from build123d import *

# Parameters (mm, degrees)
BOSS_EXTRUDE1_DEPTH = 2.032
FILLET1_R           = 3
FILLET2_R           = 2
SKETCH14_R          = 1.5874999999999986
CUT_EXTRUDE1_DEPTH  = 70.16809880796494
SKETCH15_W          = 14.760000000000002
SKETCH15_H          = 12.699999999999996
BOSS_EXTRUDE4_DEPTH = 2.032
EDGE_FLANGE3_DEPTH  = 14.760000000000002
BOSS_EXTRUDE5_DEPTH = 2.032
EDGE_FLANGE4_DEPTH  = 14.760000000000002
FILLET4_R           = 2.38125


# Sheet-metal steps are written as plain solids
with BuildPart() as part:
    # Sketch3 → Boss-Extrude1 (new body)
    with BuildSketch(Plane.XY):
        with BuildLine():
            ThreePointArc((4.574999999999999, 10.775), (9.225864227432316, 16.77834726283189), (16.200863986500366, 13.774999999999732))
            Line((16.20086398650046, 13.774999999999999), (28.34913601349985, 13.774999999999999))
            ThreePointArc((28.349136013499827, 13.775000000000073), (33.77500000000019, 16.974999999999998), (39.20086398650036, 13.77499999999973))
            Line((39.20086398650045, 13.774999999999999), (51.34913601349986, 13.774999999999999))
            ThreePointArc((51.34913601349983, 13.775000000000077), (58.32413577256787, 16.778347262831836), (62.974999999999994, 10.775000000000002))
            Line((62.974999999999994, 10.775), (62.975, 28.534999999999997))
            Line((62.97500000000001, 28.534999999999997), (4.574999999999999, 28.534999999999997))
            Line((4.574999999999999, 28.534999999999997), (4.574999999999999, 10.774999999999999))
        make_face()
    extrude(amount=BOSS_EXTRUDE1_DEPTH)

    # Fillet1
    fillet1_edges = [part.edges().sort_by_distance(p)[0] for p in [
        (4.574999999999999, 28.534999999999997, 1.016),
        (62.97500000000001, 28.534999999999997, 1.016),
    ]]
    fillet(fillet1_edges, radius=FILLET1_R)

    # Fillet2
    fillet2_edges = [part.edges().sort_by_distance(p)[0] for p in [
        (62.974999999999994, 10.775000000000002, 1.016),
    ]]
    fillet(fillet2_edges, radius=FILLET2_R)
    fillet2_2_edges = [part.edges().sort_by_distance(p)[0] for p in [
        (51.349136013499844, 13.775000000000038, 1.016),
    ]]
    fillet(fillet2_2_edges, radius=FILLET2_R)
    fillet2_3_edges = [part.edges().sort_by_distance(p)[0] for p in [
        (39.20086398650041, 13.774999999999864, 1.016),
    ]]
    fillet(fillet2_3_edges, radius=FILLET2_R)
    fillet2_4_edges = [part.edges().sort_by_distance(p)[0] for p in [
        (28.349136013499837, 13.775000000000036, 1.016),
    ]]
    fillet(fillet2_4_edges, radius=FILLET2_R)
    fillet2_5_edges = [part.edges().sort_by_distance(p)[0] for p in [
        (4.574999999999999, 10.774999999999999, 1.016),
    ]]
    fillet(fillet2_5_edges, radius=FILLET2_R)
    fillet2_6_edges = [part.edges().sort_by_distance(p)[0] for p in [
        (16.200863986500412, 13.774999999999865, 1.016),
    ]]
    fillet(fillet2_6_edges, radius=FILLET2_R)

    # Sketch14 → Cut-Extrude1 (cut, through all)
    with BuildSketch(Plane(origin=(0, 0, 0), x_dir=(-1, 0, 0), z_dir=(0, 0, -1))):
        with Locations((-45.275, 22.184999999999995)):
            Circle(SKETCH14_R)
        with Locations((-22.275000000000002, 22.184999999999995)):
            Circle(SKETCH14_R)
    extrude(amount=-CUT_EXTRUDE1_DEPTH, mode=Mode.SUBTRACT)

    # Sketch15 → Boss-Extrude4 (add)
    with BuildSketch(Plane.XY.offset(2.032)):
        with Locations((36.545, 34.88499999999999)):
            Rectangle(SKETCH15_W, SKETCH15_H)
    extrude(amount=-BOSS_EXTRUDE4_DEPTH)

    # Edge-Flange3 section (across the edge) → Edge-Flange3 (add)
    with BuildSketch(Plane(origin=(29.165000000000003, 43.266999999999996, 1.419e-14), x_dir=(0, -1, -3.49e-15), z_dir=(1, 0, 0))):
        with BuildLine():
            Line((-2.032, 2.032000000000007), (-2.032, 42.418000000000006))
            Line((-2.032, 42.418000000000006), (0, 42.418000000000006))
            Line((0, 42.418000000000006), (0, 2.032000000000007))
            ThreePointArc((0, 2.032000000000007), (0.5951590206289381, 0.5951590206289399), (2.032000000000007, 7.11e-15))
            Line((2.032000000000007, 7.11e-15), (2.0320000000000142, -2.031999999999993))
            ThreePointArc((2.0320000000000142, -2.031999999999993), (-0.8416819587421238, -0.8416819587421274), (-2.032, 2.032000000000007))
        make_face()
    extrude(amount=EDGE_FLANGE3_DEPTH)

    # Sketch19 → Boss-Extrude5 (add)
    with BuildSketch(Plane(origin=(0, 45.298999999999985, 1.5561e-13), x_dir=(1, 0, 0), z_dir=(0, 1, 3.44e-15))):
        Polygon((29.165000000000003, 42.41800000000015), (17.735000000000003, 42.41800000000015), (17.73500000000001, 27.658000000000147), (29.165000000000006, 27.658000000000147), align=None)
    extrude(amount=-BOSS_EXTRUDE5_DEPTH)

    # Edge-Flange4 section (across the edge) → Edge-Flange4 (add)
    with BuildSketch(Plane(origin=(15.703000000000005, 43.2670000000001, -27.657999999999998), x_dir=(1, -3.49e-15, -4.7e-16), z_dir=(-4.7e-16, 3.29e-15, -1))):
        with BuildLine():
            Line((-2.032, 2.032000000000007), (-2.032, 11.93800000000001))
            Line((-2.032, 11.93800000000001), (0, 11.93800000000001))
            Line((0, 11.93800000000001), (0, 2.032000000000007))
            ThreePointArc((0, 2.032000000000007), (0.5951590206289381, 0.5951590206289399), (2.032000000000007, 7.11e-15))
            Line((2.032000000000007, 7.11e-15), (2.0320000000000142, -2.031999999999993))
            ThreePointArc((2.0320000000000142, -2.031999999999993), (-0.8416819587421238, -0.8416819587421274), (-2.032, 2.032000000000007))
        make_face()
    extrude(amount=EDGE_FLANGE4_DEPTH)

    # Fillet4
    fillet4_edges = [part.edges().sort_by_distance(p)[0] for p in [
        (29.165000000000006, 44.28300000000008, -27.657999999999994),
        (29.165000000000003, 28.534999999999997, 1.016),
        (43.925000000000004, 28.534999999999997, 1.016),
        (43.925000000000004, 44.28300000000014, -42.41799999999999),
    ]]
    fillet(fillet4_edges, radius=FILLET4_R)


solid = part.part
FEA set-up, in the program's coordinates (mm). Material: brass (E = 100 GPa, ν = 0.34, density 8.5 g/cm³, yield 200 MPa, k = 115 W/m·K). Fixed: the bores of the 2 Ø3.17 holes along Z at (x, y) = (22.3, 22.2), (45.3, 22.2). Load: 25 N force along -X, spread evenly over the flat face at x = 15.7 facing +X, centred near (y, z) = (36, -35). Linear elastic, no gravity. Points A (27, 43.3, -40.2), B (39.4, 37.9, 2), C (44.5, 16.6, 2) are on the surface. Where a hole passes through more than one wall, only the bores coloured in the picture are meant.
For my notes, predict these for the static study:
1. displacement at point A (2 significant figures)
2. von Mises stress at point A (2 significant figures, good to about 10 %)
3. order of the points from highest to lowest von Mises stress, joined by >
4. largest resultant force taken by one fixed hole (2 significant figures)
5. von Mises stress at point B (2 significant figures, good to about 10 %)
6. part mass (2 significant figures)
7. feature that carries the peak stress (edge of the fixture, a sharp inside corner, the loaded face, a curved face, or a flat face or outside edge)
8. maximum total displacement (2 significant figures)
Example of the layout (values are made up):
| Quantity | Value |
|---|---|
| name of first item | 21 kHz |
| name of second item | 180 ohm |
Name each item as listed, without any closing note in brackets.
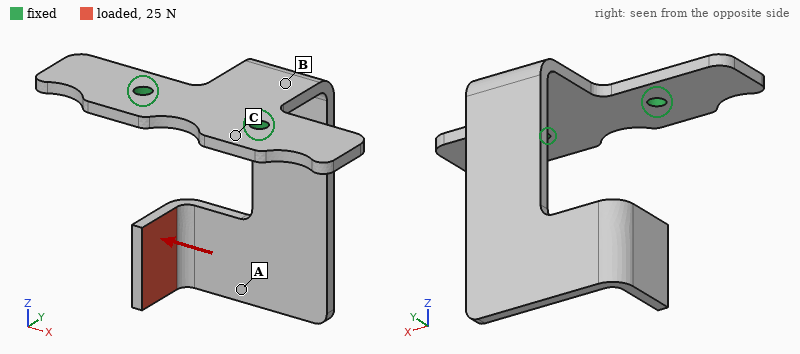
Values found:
| Quantity | Value |
|---|---|
| displacement at point A | 0.43 mm |
| von Mises stress at point A | 18 MPa |
| order of the points from highest to lowest von Mises stress, joined by > | B > A > C |
| largest resultant force taken by one fixed hole | 52 N |
| von Mises stress at point B | 73 MPa |
| part mass | 35 g |
| feature that carries the peak stress | a curved face |
| maximum total displacement | 0.62 mm |
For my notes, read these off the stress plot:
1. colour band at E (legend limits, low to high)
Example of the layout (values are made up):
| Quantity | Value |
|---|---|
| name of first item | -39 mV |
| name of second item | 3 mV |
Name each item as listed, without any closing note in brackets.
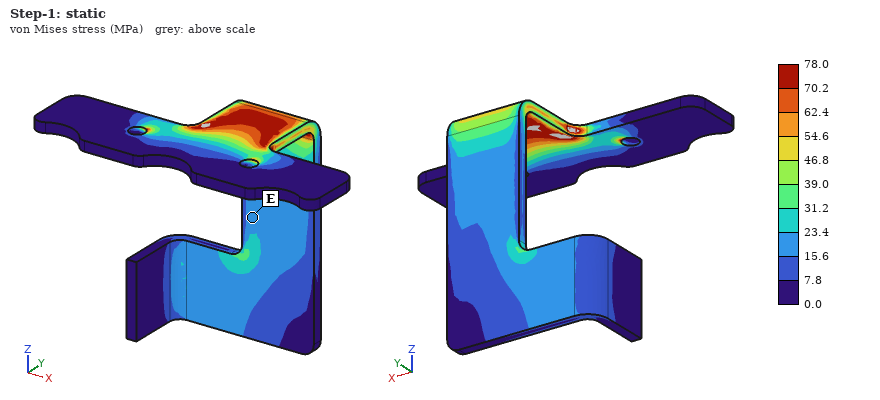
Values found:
| Quantity | Value |
|---|---|
| colour band at E | 15.6 to 23.4 MPa |
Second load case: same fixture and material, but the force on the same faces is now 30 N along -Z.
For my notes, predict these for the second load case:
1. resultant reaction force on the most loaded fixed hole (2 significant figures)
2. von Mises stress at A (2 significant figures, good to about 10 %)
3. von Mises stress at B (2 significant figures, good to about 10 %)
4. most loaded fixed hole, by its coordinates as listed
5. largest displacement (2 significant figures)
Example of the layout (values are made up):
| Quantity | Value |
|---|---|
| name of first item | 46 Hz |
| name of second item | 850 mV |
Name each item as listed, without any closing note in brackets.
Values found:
| Quantity | Value |
|---|---|
| resultant reaction force on the most loaded fixed hole | 44 N |
| von Mises stress at A | 16 MPa |
| von Mises stress at B | 49 MPa |
| most loaded fixed hole, by its coordinates as listed | (22.3, 22.2) |
| largest displacement | 0.45 mm |
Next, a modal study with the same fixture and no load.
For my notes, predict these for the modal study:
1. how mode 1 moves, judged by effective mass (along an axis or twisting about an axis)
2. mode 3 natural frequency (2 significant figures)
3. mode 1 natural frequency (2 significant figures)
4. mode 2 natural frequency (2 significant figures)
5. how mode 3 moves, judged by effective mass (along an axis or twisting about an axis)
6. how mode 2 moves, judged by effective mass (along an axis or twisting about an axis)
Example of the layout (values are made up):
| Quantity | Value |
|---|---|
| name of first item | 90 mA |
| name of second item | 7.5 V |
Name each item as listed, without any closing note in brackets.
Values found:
| Quantity | Value |
|---|---|
| how mode 1 moves, judged by effective mass | along Y |
| mode 3 natural frequency | 790 Hz |
| mode 1 natural frequency | 220 Hz |
| mode 2 natural frequency | 360 Hz |
| how mode 3 moves, judged by effective mass | along Z |
| how mode 2 moves, judged by effective mass | along X |
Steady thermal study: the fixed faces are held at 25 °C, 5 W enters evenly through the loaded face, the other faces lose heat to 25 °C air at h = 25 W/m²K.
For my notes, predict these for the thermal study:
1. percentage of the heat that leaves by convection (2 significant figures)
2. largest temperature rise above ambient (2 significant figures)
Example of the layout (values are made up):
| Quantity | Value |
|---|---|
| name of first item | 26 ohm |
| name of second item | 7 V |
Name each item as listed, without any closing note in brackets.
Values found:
| Quantity | Value |
|---|---|
| percentage of the heat that leaves by convection | 50 % |
| largest temperature rise above ambient | 74 K |
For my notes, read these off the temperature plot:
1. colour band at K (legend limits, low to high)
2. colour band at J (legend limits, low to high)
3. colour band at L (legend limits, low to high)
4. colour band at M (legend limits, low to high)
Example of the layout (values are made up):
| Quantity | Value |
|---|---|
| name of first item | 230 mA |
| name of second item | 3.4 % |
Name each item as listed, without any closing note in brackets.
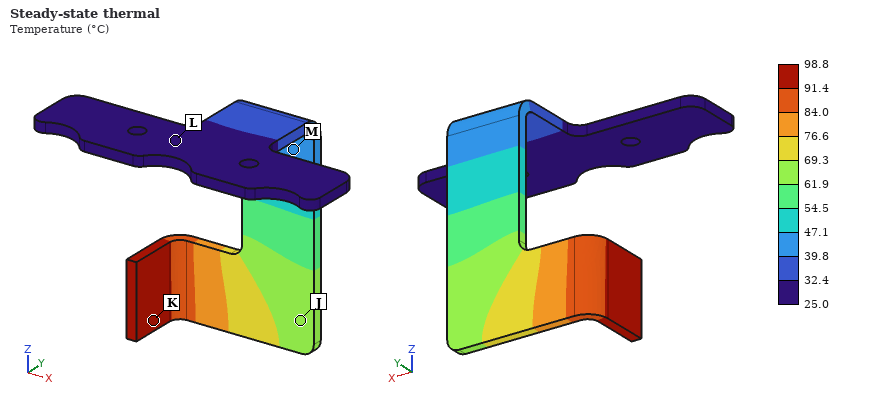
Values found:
| Quantity | Value |
|---|---|
| colour band at K | 91.4 to 98.8 °C |
| colour band at J | 61.9 to 69.3 °C |
| colour band at L | 25.0 to 32.4 °C |
| colour band at M | 39.8 to 47.1 °C |
